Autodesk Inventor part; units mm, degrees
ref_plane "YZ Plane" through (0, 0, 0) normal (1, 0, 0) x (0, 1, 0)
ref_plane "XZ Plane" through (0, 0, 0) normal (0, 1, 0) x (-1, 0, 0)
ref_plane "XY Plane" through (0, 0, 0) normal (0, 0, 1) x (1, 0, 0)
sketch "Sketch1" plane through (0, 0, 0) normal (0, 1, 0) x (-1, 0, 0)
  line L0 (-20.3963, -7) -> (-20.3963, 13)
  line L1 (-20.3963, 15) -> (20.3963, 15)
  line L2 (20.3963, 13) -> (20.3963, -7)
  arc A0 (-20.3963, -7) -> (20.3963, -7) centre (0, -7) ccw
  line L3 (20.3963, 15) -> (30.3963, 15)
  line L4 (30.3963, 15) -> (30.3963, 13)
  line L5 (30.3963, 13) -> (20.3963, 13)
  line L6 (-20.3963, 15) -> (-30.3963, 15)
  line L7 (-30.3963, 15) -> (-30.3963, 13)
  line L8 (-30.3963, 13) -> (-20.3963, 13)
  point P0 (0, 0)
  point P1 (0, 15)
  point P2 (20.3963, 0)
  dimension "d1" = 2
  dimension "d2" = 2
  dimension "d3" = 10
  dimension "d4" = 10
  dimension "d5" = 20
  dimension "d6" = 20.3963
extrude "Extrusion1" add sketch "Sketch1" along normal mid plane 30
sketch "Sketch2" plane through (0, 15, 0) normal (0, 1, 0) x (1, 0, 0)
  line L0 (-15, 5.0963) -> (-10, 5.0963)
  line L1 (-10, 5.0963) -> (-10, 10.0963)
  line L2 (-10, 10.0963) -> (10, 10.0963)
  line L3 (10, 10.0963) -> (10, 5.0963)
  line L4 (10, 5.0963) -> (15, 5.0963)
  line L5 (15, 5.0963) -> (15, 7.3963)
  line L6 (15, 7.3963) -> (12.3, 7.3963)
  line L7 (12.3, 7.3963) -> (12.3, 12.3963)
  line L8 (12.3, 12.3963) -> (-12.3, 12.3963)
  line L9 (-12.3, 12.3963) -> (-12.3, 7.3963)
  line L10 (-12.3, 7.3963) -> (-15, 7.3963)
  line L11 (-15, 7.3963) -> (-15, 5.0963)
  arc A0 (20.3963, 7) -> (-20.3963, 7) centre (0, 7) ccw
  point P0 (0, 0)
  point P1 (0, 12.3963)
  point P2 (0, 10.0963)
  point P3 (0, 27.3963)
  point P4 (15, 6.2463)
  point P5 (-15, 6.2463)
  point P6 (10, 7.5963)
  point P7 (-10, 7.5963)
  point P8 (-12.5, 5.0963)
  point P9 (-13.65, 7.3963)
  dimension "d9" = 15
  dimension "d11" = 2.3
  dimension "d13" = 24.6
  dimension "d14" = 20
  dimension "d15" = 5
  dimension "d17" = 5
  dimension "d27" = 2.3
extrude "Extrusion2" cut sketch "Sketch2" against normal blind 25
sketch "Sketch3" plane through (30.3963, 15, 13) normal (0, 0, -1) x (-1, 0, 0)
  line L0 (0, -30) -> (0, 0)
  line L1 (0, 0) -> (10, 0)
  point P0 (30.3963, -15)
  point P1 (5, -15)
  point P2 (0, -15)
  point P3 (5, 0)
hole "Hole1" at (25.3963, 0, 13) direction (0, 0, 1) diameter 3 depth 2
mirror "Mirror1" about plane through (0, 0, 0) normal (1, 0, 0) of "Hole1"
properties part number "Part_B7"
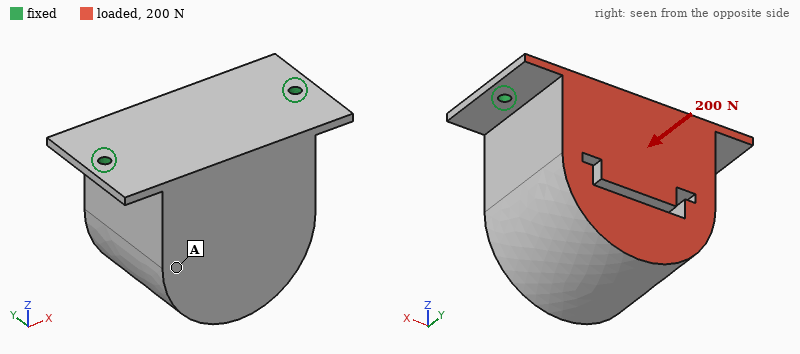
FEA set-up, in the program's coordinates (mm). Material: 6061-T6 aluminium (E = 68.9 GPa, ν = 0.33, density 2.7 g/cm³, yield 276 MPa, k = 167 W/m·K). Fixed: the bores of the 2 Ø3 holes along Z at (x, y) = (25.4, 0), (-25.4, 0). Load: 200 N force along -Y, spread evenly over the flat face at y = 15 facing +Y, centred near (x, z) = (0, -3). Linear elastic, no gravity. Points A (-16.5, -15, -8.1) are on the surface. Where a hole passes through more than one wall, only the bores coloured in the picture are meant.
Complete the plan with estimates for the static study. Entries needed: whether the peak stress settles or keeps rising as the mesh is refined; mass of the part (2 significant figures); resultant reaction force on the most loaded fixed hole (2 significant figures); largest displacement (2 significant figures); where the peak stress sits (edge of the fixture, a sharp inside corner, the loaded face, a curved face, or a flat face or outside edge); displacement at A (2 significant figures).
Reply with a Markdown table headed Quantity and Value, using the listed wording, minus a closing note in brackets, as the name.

| Quantity | Value |
|---|---|
| whether the peak stress settles or keeps rising as the mesh is refined | keeps rising |
| mass of the part | 120 g |
| resultant reaction force on the most loaded fixed hole | 100 N |
| largest displacement | 0.21 mm |
| where the peak stress sits | edge of the fixture |
| displacement at A | 0.13 mm |
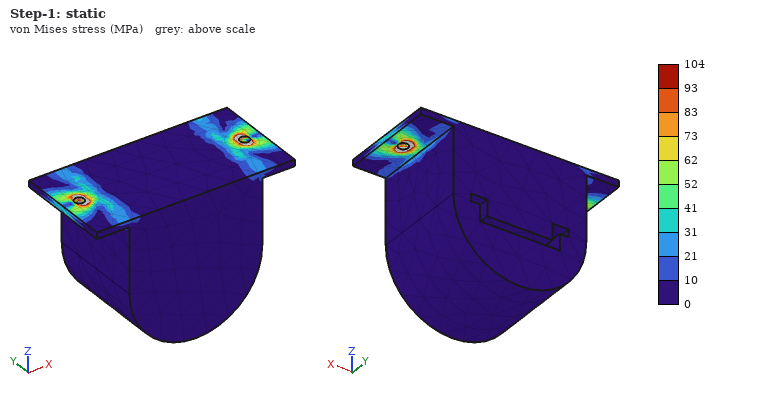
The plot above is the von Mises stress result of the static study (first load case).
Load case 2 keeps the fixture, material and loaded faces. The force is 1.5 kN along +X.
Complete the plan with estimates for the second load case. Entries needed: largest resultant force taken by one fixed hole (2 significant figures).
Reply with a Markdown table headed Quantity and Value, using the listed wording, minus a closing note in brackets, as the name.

| Quantity | Value |
|---|---|
| largest resultant force taken by one fixed hole | 1.0 kN |
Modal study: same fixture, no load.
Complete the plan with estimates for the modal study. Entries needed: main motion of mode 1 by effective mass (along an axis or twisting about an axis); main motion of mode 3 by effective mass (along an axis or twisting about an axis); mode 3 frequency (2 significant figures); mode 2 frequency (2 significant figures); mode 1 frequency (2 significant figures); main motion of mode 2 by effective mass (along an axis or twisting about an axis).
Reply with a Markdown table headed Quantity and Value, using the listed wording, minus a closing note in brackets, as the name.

| Quantity | Value |
|---|---|
| main motion of mode 1 by effective mass | along Y |
| main motion of mode 3 by effective mass | along Z |
| mode 3 frequency | 3400 Hz |
| mode 2 frequency | 3200 Hz |
| mode 1 frequency | 530 Hz |
| main motion of mode 2 by effective mass | along X |
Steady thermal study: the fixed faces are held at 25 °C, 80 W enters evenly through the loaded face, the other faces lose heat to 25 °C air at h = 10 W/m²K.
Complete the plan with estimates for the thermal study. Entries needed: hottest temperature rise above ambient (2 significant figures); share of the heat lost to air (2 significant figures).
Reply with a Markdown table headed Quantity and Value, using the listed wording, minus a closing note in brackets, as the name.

| Quantity | Value |
|---|---|
| hottest temperature rise above ambient | 62 K |
| share of the heat lost to air | 5.9 % |
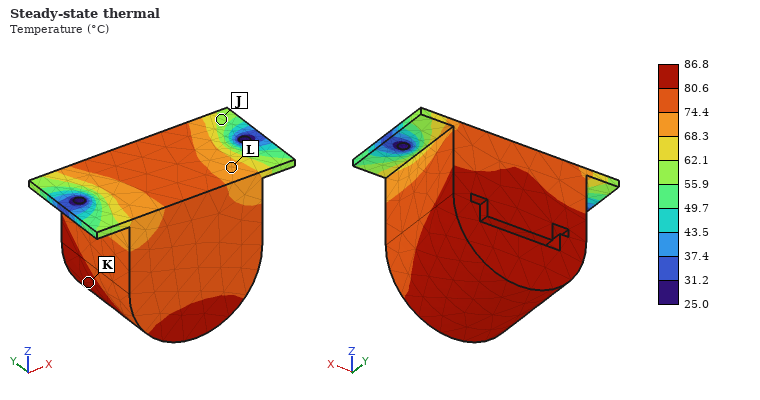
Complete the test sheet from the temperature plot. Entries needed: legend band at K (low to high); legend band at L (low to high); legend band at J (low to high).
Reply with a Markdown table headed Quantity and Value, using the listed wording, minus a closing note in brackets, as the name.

| Quantity | Value |
|---|---|
| legend band at K | 80.6 to 86.8 °C |
| legend band at L | 68.3 to 74.4 °C |
| legend band at J | 55.9 to 62.1 °C |
